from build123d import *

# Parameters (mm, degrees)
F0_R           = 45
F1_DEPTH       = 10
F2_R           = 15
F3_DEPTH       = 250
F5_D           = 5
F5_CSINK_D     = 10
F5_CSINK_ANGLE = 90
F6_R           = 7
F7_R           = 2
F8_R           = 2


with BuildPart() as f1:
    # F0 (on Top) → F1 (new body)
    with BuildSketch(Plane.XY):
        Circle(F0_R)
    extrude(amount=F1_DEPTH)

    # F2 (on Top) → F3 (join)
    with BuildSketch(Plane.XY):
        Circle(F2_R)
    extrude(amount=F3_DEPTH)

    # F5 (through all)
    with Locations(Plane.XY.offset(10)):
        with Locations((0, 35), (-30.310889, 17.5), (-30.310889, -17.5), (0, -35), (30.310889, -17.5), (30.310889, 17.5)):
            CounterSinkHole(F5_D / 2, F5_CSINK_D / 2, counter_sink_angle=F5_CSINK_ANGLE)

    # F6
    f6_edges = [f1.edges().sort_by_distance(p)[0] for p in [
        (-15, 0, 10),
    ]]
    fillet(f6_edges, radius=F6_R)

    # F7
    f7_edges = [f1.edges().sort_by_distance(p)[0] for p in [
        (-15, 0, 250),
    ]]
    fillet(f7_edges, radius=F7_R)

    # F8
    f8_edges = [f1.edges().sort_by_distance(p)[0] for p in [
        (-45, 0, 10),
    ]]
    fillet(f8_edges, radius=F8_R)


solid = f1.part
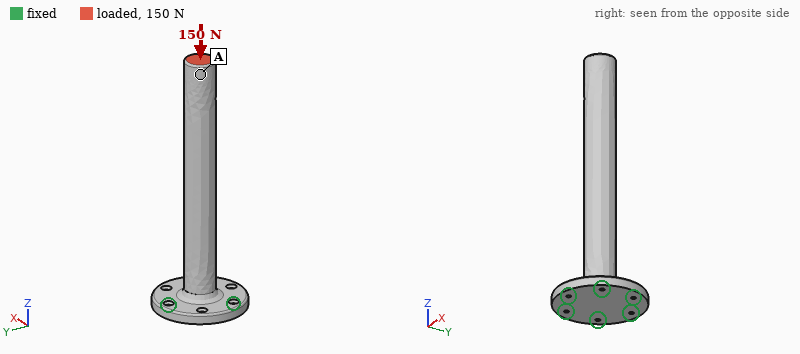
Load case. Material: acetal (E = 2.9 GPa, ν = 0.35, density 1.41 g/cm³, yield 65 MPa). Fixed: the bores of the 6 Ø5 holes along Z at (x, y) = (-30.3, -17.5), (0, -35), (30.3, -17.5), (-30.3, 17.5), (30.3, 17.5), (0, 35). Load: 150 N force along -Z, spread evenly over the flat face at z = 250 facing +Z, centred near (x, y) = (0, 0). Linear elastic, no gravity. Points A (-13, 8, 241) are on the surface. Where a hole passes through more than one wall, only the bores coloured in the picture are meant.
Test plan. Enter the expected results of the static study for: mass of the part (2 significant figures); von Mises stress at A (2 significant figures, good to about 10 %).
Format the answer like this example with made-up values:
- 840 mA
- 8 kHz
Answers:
- 330 g
- 0.18 MPa
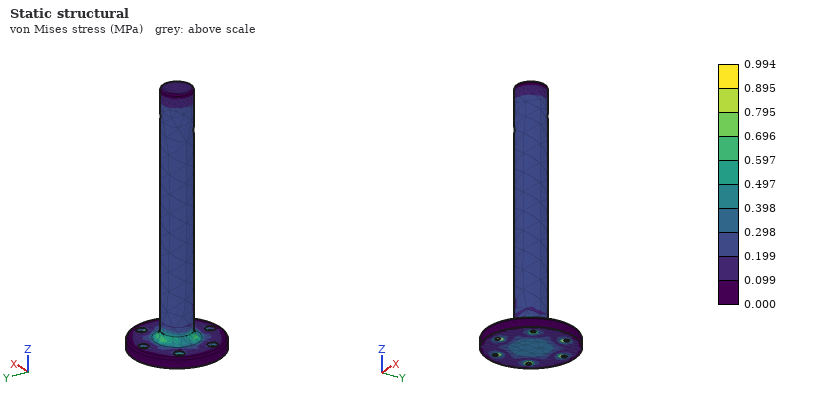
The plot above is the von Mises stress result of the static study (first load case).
